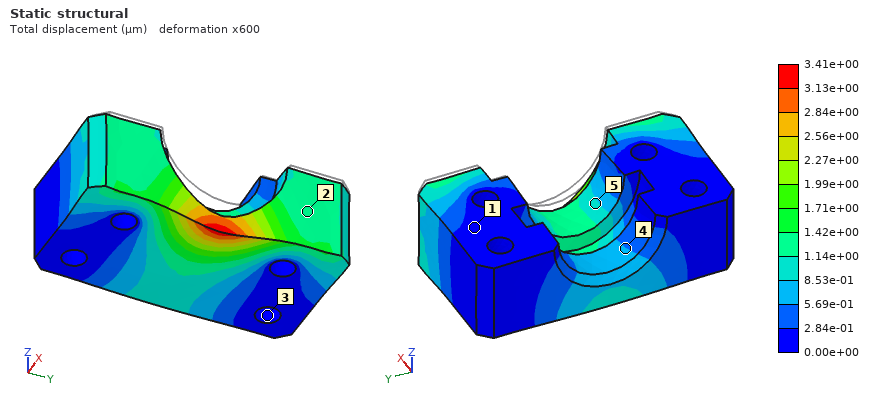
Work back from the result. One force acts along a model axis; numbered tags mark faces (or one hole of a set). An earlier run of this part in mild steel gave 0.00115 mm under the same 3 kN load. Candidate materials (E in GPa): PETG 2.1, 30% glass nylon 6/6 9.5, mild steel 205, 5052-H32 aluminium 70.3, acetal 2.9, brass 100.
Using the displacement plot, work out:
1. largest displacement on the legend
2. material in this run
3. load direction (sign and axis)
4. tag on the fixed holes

3.41e+00 µm
5052-H32 aluminium
-X
3
